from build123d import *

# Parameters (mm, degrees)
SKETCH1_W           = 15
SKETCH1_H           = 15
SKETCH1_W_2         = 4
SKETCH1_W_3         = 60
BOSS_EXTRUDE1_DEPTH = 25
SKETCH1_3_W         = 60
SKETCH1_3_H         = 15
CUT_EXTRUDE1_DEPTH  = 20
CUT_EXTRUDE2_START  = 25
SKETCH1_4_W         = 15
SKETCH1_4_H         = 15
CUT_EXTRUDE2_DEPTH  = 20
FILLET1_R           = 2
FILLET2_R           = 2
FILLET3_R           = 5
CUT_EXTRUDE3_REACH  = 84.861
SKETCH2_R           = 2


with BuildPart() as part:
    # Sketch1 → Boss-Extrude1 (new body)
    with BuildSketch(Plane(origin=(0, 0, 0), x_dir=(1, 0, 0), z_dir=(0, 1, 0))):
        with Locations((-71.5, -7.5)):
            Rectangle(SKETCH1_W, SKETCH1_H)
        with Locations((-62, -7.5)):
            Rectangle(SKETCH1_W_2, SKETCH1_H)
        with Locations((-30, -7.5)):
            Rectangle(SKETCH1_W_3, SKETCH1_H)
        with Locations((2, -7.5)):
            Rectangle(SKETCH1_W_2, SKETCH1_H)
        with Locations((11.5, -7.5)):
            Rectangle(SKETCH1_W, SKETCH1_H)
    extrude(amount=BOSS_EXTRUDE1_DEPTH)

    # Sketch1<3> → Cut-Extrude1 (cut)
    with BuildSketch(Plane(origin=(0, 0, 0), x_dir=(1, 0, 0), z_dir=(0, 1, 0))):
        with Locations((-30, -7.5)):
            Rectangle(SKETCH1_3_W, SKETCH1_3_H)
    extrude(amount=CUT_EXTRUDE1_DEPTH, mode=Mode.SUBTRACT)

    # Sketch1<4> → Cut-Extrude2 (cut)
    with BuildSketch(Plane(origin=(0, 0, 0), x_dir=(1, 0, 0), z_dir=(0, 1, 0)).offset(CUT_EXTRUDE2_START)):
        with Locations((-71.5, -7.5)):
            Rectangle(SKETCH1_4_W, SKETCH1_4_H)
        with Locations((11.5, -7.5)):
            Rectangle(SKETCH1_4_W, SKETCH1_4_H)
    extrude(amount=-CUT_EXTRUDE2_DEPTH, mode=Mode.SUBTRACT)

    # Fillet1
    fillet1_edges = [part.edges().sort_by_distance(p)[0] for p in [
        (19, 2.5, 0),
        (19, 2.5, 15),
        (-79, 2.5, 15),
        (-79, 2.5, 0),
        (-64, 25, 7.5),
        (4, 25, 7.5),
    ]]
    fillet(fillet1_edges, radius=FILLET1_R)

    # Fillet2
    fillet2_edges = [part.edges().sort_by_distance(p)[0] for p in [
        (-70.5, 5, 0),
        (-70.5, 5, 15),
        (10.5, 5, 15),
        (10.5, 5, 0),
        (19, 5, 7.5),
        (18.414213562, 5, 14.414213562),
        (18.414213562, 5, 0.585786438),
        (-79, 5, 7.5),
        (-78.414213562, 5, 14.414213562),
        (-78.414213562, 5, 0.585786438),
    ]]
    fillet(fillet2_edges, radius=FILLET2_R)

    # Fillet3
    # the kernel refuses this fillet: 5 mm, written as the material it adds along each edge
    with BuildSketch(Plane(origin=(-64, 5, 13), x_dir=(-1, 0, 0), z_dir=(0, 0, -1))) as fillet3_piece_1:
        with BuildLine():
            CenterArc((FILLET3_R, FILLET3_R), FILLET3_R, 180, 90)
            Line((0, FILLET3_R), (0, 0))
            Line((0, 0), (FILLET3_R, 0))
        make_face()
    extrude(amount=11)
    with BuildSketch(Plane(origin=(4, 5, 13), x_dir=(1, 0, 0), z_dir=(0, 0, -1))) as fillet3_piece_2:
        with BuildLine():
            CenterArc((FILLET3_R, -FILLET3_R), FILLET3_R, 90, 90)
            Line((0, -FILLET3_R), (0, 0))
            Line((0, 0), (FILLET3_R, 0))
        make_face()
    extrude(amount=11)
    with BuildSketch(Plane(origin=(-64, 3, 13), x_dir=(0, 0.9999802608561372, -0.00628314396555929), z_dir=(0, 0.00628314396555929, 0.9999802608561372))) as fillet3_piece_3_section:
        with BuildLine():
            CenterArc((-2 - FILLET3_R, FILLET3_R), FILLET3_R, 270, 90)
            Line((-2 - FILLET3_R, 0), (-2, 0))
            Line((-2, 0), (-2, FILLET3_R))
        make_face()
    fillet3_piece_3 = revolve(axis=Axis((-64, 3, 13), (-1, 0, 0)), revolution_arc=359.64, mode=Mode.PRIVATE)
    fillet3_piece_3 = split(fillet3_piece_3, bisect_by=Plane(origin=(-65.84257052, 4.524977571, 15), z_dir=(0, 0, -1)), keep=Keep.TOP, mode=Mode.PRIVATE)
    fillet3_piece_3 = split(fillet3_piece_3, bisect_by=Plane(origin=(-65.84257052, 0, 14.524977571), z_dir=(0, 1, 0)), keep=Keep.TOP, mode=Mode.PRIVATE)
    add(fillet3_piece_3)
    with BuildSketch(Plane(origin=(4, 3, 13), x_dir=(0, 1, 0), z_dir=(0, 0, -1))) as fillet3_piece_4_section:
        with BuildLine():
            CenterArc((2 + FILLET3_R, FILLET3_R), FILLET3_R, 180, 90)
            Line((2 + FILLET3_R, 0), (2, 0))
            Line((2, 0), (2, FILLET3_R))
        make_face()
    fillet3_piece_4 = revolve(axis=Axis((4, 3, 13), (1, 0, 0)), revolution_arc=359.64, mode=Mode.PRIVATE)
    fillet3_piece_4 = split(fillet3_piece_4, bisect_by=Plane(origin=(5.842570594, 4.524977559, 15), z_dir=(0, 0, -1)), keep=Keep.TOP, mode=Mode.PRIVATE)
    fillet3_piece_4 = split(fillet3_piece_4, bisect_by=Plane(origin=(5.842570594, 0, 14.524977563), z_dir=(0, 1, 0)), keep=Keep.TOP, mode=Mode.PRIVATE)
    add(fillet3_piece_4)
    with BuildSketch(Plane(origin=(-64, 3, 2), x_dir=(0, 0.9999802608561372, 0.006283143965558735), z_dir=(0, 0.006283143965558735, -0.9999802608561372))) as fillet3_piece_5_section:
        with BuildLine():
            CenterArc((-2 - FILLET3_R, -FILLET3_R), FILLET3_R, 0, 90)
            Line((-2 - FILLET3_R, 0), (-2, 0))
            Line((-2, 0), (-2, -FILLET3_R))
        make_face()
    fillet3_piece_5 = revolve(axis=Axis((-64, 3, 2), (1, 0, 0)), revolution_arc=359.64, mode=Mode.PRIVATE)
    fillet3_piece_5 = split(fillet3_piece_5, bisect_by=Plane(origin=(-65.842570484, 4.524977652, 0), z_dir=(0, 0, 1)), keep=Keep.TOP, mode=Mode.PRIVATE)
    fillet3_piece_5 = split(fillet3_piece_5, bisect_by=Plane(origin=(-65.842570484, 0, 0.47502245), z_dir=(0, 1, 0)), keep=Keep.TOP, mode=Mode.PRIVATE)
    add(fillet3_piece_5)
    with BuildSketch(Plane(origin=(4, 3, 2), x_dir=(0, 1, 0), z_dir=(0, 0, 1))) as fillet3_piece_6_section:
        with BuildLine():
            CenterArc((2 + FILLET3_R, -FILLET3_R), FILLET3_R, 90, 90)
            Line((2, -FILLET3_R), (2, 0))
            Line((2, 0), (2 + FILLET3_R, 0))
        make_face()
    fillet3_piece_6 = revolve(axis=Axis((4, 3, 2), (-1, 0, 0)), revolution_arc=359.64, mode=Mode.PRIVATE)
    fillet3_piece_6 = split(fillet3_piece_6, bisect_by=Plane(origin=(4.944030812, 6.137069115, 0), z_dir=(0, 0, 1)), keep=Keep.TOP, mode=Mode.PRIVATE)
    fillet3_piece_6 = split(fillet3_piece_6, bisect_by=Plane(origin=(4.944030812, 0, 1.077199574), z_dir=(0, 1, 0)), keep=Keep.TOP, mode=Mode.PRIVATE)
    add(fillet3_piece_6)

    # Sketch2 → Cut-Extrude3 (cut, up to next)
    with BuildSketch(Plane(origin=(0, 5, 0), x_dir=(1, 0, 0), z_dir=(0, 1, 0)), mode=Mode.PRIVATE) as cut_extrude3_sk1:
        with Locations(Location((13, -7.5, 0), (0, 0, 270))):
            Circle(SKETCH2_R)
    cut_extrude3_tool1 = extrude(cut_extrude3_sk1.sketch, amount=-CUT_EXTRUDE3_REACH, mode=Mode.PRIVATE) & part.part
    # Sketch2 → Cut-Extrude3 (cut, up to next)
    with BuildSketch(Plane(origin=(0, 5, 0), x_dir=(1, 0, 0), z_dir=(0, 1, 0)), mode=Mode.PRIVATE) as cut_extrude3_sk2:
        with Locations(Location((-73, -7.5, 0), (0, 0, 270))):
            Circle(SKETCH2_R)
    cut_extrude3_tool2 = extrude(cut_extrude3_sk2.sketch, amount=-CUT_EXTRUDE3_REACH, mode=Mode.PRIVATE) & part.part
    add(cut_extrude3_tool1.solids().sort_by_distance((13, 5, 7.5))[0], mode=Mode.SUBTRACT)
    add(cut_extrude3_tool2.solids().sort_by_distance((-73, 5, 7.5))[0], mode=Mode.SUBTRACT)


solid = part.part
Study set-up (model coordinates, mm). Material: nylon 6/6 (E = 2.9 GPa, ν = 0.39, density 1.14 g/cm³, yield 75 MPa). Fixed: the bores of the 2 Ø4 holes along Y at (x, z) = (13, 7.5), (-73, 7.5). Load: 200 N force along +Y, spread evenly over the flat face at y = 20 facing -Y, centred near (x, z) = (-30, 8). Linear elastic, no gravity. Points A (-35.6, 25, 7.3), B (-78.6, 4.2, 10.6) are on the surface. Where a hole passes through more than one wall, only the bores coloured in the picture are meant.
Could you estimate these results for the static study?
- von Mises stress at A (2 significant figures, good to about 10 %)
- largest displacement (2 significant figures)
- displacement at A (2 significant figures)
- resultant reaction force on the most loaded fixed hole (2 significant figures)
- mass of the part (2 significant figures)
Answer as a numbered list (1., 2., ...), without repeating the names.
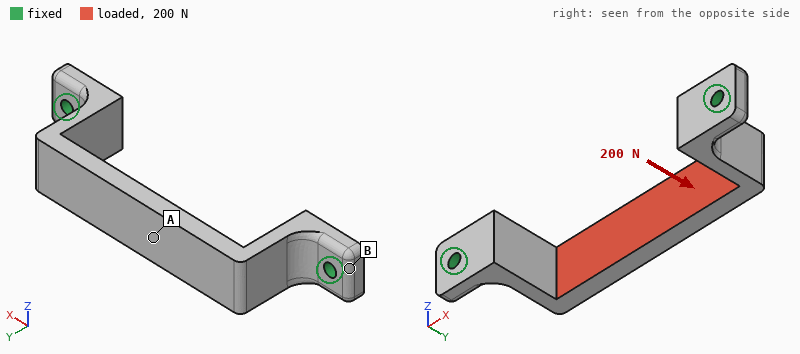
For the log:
1. 12 MPa
2. 0.57 mm
3. 0.52 mm
4. 130 N
5. 11 g
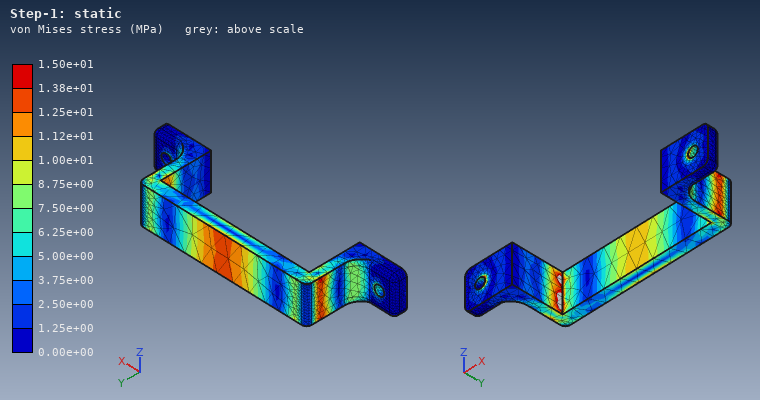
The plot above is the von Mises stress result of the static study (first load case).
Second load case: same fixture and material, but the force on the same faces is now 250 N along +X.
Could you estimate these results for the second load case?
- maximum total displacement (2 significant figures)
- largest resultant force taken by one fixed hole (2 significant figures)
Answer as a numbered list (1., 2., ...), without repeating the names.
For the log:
1. 0.65 mm
2. 130 N
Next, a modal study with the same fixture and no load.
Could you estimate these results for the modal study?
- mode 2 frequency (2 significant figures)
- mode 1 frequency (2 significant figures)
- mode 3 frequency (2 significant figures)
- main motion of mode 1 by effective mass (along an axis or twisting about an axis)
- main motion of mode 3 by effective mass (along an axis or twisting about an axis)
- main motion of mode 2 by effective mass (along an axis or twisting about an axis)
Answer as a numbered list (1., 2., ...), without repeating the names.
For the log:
1. 1200 Hz
2. 1000 Hz
3. 1500 Hz
4. along Z
5. along Y
6. along X
